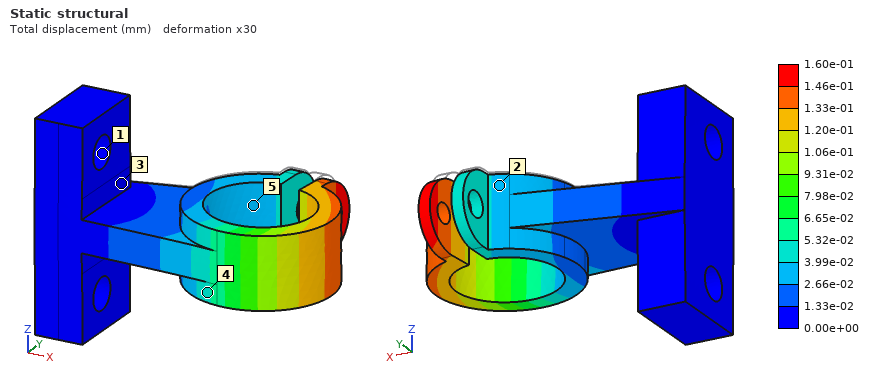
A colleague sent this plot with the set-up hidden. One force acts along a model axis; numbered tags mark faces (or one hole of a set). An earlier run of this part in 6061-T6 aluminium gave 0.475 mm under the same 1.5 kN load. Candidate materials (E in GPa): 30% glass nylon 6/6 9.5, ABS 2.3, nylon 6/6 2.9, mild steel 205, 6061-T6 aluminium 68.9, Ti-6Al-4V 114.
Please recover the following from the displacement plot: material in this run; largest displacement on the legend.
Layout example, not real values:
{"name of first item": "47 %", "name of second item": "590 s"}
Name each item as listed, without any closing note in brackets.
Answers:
{"material in this run": "mild steel", "largest displacement on the legend": "1.60e-01 mm"}
